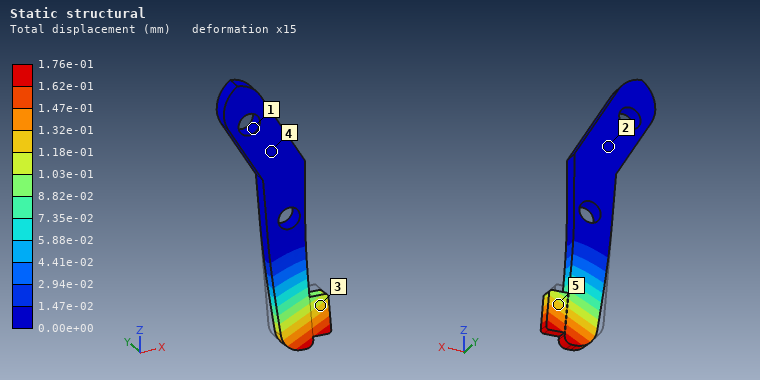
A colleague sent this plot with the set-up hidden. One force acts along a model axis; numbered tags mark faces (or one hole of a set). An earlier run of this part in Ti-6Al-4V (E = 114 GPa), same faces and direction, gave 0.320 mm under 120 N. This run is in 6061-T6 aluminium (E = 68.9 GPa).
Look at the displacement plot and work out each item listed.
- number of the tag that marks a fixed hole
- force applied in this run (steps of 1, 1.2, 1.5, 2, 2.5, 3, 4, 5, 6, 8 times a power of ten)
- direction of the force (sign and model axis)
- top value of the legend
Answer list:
1
40 N
-Y
1.76e-01 mm
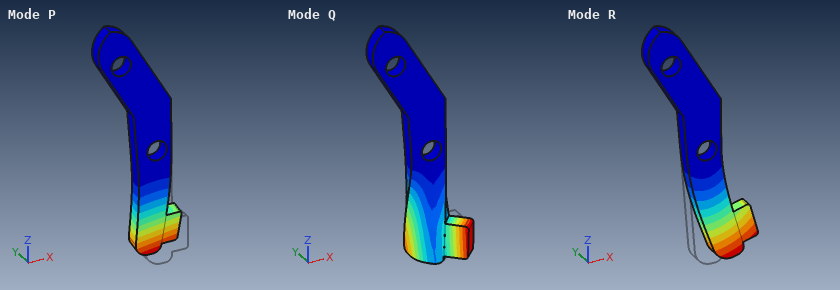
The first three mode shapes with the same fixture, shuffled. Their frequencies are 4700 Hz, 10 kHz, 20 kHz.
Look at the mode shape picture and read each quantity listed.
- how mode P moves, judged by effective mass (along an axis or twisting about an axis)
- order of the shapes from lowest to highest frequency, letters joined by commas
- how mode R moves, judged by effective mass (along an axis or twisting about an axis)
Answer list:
along Y
P, R, Q
along X
